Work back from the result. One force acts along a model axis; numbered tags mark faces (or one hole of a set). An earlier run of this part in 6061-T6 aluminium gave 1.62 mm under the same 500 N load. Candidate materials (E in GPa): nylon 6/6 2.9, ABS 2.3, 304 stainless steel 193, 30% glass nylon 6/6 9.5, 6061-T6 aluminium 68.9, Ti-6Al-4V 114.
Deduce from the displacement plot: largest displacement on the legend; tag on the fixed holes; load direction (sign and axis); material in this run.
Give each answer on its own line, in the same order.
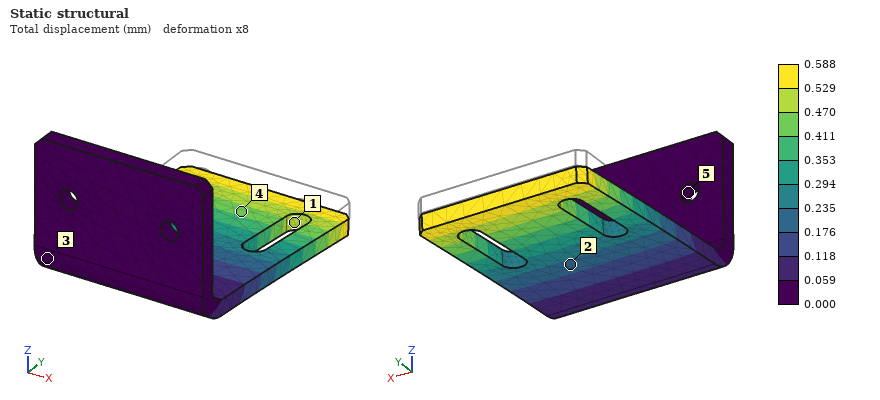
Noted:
0.588 mm
5
-Z
304 stainless steel
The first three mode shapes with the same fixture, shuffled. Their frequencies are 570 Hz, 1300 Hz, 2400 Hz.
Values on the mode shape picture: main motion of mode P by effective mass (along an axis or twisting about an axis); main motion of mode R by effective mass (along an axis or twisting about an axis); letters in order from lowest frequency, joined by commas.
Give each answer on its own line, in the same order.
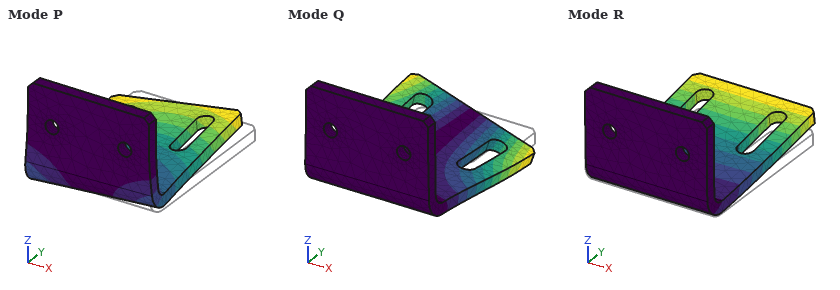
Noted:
along X
along Z
R, P, Q
